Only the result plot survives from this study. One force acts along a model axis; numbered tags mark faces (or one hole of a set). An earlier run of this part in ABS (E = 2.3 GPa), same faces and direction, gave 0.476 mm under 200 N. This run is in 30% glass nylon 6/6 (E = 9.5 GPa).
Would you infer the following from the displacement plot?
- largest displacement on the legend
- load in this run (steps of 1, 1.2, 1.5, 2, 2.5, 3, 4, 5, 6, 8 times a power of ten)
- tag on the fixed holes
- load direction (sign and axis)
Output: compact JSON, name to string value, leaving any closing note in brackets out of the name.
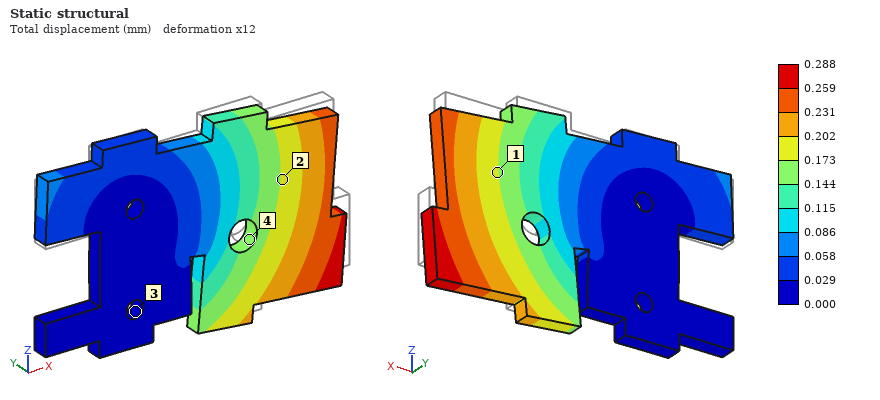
{"largest displacement on the legend": "0.288 mm", "load in this run": "500 N", "tag on the fixed holes": "3", "load direction": "-Z"}
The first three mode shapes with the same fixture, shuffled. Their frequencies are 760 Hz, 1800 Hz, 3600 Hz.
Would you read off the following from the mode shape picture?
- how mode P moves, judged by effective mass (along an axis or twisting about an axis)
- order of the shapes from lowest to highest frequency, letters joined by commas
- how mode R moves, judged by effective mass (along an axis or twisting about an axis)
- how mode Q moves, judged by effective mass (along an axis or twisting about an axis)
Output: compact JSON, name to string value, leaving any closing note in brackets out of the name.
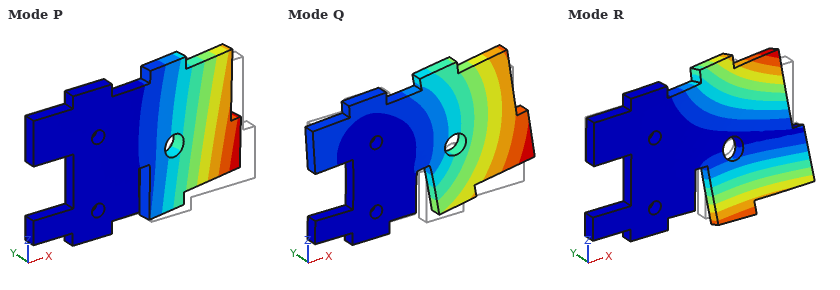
{"how mode P moves, judged by effective mass": "along Y", "order of the shapes from lowest to highest frequency, letters joined by commas": "P, R, Q", "how mode R moves, judged by effective mass": "twisting about X", "how mode Q moves, judged by effective mass": "along Z"}
